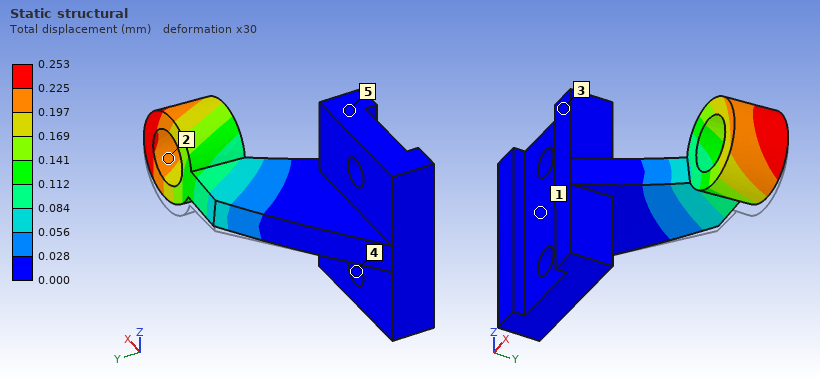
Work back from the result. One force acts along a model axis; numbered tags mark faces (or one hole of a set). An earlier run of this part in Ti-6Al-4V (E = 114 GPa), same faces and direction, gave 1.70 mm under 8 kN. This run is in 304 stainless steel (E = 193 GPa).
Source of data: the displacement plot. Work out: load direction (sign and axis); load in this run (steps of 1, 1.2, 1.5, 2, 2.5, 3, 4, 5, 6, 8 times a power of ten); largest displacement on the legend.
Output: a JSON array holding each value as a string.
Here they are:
["+Z", "2 kN", "0.253 mm"]
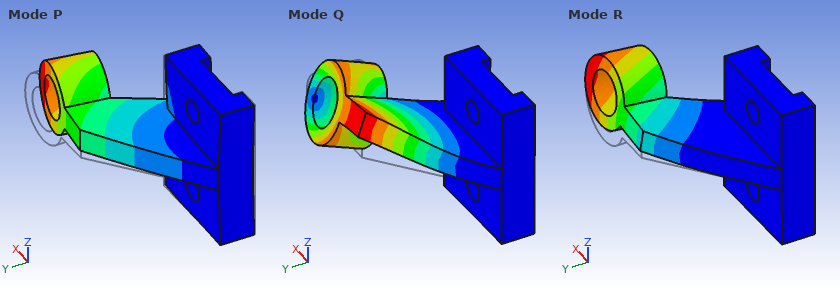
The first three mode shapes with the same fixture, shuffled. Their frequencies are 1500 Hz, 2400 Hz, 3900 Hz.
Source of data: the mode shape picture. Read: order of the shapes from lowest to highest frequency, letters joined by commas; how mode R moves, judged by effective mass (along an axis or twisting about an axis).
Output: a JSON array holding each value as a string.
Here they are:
["R, P, Q", "along Z"]
